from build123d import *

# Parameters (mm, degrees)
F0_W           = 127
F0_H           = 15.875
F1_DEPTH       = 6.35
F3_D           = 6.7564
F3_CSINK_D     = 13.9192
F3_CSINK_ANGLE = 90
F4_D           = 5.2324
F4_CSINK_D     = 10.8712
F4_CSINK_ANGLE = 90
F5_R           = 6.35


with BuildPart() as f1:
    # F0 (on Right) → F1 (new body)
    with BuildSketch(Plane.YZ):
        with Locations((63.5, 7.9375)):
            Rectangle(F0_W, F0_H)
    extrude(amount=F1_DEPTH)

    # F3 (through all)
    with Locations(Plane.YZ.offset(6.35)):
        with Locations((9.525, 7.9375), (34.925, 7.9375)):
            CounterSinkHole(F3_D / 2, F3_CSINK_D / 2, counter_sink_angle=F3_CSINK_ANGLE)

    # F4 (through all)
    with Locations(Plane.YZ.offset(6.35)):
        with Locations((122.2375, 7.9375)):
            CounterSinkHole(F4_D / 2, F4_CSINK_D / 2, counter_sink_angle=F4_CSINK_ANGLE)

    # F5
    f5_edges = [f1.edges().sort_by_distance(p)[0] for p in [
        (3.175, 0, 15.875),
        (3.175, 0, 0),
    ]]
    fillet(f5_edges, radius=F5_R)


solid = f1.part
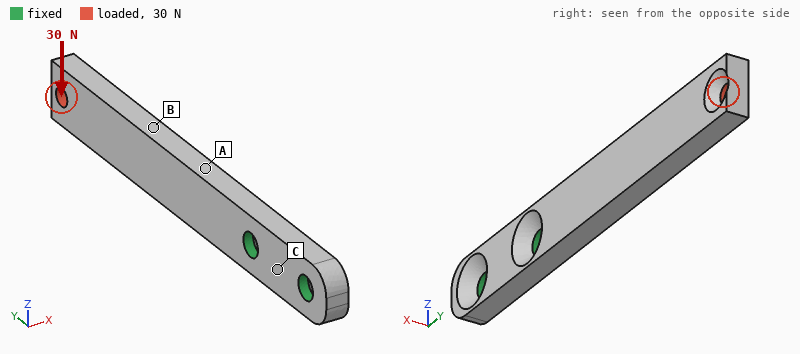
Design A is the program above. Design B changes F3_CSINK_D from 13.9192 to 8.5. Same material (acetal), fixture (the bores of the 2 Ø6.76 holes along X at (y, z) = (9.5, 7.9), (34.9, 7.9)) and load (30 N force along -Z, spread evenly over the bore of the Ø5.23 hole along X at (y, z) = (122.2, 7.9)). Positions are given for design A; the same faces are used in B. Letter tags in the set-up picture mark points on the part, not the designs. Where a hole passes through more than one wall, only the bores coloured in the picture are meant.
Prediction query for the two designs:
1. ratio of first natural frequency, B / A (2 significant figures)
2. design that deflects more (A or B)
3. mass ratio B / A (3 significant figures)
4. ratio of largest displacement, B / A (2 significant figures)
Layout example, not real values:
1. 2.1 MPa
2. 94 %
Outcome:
1. 1.1
2. A
3. 1.03
4. 0.91
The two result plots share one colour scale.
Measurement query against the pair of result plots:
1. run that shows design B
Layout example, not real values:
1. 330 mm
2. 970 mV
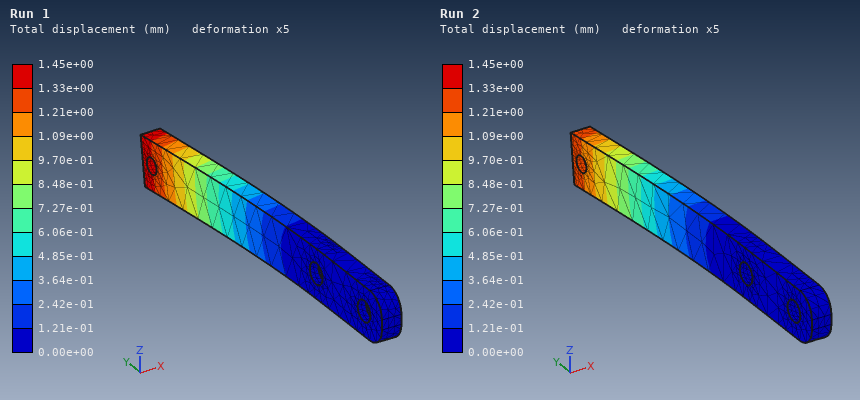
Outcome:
1. Run 2
